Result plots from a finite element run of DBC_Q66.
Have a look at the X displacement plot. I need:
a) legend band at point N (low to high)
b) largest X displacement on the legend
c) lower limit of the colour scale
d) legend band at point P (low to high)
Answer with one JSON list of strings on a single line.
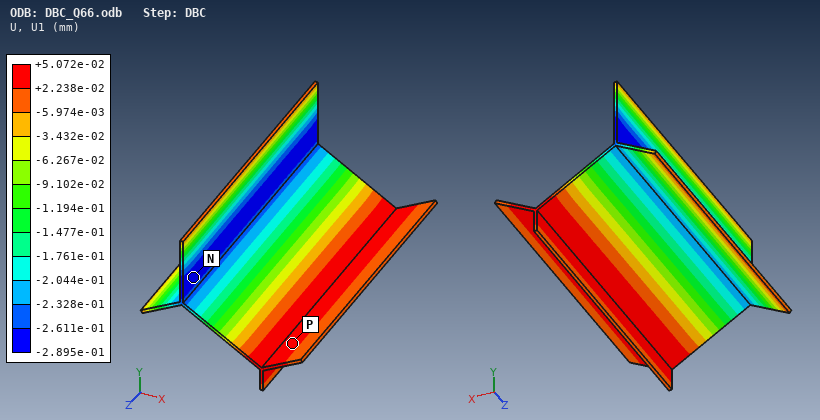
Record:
["-2.895e-01 to -2.611e-01 mm", "+5.072e-02 mm", "-2.895e-01 mm", "+2.238e-02 to +5.072e-02 mm"]
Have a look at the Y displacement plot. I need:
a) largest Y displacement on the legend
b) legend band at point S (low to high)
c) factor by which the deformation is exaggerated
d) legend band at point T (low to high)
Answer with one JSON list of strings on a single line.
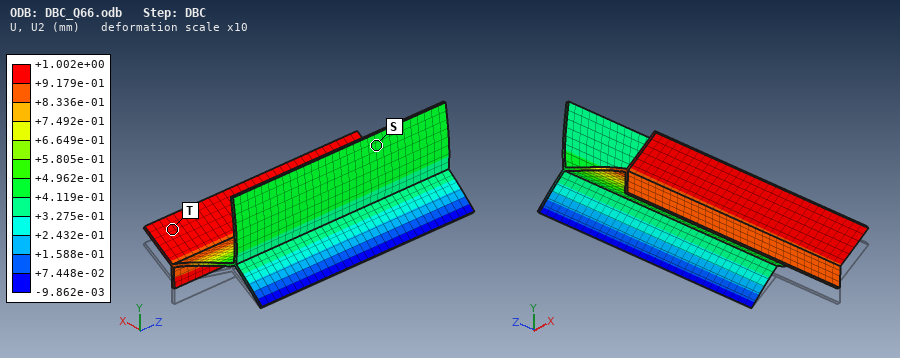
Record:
["+1.002e+00 mm", "+4.119e-01 to +4.962e-01 mm", "10", "+9.179e-01 to +1.002e+00 mm"]
